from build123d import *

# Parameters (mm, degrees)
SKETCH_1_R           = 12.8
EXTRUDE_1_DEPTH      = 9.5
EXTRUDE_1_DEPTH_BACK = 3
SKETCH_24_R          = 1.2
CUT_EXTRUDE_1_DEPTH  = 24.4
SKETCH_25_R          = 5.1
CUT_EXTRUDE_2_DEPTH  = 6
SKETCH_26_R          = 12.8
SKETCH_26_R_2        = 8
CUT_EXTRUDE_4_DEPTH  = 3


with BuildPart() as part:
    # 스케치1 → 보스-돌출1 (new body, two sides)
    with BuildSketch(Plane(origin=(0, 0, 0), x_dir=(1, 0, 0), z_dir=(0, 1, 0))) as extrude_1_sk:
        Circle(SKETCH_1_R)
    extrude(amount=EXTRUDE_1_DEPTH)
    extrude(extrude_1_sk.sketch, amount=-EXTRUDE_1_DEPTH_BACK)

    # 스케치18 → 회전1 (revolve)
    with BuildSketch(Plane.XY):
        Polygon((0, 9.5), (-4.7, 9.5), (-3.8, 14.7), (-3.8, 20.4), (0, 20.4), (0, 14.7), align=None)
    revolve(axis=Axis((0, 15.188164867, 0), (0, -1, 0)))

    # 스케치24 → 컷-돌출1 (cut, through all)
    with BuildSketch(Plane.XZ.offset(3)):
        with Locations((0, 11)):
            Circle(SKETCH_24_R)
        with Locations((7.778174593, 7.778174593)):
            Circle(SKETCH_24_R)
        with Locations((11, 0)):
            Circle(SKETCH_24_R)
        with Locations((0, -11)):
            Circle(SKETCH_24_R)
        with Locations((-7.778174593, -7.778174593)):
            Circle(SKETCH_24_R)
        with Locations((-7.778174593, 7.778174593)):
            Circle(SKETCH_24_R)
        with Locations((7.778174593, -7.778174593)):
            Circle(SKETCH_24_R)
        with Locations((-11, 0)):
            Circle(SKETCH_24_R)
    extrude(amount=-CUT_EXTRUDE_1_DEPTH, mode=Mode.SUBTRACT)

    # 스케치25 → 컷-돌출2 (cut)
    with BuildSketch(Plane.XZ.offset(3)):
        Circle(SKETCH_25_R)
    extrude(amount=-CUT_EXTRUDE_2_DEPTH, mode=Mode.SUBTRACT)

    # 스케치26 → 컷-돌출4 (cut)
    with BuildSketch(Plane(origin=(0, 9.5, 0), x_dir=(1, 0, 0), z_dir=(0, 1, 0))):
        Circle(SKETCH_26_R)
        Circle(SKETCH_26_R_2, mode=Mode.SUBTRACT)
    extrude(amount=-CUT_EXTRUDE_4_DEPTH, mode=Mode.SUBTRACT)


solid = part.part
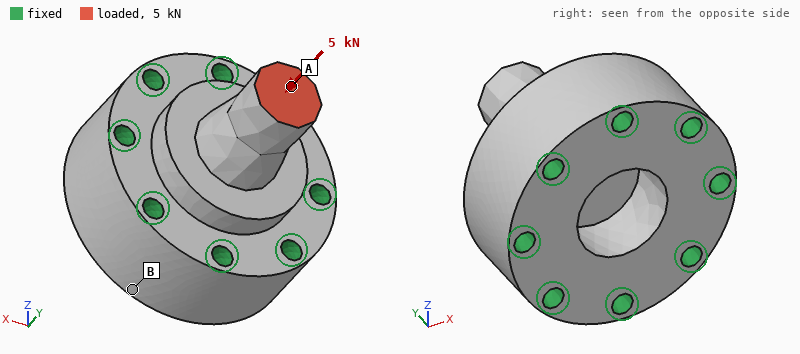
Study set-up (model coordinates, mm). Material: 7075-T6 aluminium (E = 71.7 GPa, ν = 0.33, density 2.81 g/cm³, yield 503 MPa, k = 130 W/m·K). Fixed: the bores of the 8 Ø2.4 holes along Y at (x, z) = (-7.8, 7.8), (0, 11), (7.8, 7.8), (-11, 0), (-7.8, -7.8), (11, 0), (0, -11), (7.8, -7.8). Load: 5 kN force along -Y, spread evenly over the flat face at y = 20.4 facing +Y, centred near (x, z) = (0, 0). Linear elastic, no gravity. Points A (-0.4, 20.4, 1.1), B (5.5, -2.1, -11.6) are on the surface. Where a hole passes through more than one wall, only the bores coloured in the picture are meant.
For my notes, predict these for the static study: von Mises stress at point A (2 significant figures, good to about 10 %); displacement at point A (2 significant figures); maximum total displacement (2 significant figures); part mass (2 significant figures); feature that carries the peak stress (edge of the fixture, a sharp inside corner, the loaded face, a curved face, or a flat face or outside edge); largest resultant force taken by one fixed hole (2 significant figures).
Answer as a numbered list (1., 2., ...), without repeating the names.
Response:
1. 110 MPa
2. 21 µm
3. 21 µm
4. 15 g
5. a sharp inside corner
6. 800 N
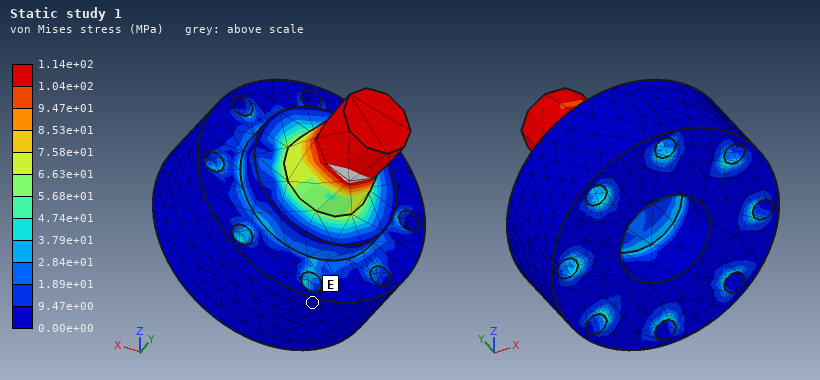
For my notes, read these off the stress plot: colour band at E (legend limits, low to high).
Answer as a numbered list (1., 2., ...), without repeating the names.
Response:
1. 0.00e+00 to 9.47e+00 MPa
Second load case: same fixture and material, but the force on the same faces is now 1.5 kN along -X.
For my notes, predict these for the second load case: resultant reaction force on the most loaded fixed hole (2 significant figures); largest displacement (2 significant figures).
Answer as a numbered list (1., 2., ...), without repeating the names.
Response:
1. 790 N
2. 73 µm
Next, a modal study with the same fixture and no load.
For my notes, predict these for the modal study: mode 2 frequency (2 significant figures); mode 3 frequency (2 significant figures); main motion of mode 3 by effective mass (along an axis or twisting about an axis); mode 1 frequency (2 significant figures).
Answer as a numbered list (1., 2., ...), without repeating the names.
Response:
1. 35 kHz
2. 72 kHz
3. along Y
4. 35 kHz
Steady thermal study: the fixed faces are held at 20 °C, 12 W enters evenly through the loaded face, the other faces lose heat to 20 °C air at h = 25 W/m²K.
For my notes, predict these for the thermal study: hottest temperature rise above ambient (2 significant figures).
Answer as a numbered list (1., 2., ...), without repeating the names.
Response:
1. 25 K
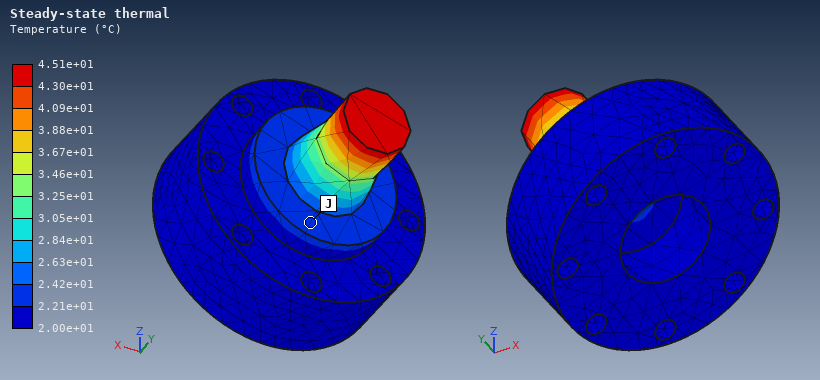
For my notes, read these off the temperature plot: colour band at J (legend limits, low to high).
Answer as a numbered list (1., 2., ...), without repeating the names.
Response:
1. 2.21e+01 to 2.42e+01 °C
